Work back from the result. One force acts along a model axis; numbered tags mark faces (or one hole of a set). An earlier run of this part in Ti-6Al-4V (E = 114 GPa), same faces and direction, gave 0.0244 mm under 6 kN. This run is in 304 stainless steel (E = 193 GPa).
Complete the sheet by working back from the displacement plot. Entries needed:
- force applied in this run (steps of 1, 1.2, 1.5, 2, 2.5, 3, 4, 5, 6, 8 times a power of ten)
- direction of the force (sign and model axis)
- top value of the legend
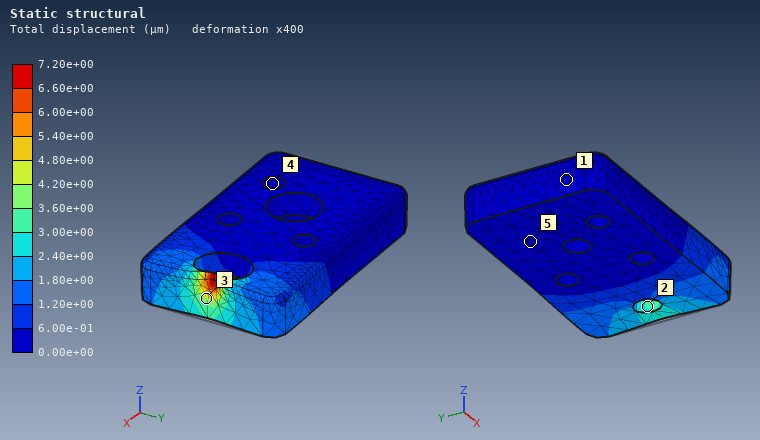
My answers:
3 kN
-X
7.20e+00 µm
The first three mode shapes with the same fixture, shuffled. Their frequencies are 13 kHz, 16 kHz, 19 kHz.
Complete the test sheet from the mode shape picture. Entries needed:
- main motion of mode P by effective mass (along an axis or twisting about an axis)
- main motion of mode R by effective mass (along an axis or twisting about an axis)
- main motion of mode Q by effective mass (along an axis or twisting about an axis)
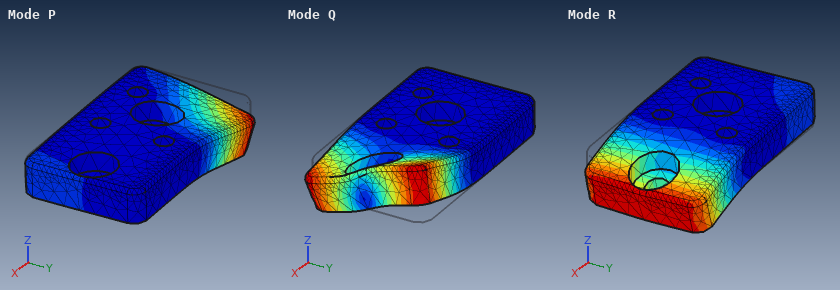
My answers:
along Z
along Z
twisting about X
